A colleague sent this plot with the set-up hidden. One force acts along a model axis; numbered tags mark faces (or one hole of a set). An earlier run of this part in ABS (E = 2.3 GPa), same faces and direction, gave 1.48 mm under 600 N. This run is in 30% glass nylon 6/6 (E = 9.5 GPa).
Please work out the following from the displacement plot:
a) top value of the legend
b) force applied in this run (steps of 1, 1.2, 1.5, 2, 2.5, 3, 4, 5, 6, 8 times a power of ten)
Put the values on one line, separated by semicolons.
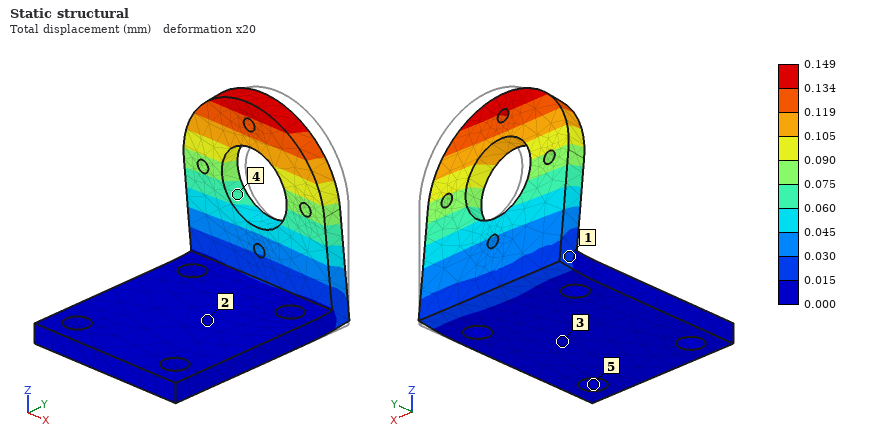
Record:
0.149 mm; 250 N
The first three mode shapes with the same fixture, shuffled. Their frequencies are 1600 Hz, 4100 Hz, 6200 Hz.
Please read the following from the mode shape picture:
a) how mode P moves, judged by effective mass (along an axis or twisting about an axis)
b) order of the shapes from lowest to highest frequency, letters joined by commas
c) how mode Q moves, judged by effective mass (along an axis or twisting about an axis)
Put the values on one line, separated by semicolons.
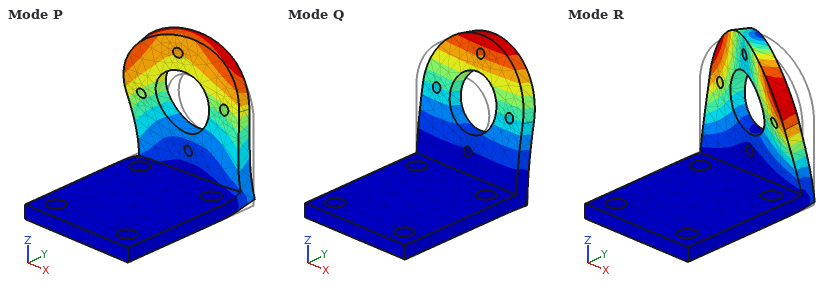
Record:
along X; Q, R, P; along Y
